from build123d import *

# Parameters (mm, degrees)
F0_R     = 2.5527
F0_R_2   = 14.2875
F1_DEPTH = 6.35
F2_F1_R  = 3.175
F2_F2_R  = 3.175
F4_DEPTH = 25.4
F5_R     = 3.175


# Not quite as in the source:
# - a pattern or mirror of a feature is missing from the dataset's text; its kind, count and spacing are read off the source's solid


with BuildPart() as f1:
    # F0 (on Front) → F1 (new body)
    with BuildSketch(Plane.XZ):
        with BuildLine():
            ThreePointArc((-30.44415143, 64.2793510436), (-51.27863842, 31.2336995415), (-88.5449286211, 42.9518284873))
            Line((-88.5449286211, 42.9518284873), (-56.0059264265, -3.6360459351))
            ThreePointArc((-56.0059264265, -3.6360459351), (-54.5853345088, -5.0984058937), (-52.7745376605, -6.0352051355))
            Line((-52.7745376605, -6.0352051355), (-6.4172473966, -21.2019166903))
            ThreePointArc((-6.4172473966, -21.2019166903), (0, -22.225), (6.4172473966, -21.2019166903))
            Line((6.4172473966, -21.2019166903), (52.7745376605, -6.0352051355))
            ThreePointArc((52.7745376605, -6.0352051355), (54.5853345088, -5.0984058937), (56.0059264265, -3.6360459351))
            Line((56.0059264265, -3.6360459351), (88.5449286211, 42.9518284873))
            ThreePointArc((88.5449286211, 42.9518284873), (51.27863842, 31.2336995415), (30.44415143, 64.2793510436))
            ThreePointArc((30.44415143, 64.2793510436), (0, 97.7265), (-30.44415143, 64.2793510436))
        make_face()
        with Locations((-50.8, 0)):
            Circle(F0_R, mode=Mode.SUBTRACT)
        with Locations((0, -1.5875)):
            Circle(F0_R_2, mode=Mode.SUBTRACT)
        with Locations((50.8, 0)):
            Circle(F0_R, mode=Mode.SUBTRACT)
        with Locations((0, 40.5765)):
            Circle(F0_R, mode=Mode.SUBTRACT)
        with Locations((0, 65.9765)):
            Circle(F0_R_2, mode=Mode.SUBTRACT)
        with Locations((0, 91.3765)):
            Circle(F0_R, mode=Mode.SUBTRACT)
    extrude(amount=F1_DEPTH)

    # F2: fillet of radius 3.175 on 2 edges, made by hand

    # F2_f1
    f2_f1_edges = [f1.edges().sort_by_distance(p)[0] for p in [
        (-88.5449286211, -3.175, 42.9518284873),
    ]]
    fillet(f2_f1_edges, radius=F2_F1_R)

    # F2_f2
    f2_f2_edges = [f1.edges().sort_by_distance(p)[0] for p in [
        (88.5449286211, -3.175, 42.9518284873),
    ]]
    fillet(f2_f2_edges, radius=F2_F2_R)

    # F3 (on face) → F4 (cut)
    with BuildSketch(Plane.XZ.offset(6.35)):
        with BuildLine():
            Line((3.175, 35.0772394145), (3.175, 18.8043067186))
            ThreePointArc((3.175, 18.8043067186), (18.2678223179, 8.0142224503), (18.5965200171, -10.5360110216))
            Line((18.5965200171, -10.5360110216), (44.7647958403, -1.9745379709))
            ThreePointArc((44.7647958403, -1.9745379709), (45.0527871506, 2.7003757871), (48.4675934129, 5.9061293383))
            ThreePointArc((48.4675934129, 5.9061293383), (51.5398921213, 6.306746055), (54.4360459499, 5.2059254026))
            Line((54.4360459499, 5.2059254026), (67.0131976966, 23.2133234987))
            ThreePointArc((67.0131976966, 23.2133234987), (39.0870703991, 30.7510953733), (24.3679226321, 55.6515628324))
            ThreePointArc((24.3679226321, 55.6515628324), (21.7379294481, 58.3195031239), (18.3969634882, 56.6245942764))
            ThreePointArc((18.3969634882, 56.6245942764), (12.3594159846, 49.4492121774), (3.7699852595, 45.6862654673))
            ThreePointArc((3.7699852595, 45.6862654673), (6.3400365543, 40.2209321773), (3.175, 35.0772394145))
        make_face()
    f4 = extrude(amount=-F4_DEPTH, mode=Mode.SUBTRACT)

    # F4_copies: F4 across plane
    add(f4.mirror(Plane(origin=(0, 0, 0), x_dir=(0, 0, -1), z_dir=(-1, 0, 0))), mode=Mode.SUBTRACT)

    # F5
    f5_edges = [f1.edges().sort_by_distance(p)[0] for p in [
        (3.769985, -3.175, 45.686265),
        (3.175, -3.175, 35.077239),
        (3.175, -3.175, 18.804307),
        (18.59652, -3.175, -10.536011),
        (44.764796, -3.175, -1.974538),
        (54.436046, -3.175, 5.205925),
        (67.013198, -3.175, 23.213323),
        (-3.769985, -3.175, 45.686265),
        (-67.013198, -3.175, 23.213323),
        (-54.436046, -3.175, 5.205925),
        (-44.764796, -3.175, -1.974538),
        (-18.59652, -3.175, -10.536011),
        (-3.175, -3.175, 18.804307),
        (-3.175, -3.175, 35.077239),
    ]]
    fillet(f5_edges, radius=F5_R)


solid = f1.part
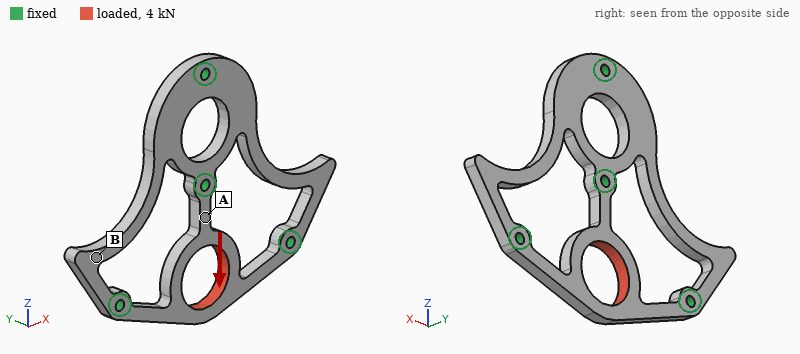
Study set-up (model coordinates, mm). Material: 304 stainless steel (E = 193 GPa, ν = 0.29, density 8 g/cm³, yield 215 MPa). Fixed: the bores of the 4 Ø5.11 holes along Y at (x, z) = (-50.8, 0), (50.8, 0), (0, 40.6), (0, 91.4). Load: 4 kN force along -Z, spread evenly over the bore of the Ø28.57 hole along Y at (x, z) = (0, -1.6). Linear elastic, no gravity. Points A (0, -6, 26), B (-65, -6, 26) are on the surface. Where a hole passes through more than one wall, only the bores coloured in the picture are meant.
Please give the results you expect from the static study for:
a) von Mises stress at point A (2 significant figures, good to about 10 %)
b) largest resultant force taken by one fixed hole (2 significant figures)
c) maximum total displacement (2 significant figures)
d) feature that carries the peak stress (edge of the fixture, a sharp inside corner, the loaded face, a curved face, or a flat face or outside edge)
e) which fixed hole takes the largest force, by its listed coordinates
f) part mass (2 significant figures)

71 MPa
2.8 kN
34 µm
a curved face
(0, 40.6)
230 g
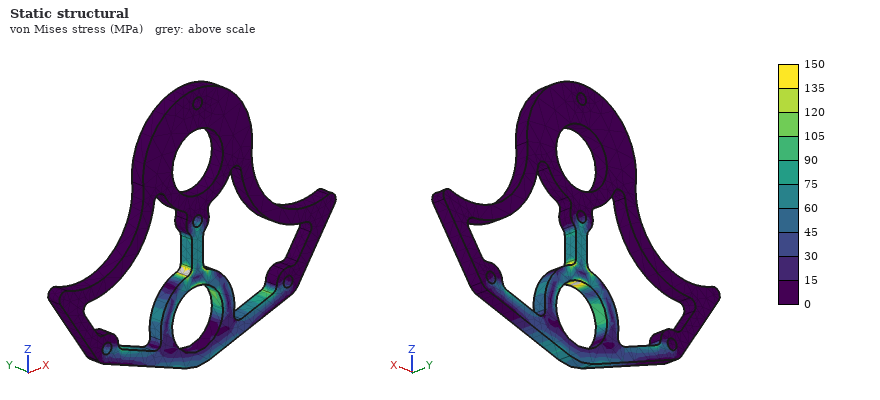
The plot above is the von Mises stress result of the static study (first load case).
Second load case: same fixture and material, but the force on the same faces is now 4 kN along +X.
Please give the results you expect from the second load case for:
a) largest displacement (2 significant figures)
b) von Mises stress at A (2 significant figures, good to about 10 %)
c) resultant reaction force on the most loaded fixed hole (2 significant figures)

46 µm
83 MPa
1.5 kN
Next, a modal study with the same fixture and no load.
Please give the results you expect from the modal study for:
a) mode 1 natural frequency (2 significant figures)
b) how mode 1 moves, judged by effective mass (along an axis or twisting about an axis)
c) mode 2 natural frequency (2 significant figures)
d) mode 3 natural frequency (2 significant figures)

2500 Hz
along Y
2700 Hz
2800 Hz
